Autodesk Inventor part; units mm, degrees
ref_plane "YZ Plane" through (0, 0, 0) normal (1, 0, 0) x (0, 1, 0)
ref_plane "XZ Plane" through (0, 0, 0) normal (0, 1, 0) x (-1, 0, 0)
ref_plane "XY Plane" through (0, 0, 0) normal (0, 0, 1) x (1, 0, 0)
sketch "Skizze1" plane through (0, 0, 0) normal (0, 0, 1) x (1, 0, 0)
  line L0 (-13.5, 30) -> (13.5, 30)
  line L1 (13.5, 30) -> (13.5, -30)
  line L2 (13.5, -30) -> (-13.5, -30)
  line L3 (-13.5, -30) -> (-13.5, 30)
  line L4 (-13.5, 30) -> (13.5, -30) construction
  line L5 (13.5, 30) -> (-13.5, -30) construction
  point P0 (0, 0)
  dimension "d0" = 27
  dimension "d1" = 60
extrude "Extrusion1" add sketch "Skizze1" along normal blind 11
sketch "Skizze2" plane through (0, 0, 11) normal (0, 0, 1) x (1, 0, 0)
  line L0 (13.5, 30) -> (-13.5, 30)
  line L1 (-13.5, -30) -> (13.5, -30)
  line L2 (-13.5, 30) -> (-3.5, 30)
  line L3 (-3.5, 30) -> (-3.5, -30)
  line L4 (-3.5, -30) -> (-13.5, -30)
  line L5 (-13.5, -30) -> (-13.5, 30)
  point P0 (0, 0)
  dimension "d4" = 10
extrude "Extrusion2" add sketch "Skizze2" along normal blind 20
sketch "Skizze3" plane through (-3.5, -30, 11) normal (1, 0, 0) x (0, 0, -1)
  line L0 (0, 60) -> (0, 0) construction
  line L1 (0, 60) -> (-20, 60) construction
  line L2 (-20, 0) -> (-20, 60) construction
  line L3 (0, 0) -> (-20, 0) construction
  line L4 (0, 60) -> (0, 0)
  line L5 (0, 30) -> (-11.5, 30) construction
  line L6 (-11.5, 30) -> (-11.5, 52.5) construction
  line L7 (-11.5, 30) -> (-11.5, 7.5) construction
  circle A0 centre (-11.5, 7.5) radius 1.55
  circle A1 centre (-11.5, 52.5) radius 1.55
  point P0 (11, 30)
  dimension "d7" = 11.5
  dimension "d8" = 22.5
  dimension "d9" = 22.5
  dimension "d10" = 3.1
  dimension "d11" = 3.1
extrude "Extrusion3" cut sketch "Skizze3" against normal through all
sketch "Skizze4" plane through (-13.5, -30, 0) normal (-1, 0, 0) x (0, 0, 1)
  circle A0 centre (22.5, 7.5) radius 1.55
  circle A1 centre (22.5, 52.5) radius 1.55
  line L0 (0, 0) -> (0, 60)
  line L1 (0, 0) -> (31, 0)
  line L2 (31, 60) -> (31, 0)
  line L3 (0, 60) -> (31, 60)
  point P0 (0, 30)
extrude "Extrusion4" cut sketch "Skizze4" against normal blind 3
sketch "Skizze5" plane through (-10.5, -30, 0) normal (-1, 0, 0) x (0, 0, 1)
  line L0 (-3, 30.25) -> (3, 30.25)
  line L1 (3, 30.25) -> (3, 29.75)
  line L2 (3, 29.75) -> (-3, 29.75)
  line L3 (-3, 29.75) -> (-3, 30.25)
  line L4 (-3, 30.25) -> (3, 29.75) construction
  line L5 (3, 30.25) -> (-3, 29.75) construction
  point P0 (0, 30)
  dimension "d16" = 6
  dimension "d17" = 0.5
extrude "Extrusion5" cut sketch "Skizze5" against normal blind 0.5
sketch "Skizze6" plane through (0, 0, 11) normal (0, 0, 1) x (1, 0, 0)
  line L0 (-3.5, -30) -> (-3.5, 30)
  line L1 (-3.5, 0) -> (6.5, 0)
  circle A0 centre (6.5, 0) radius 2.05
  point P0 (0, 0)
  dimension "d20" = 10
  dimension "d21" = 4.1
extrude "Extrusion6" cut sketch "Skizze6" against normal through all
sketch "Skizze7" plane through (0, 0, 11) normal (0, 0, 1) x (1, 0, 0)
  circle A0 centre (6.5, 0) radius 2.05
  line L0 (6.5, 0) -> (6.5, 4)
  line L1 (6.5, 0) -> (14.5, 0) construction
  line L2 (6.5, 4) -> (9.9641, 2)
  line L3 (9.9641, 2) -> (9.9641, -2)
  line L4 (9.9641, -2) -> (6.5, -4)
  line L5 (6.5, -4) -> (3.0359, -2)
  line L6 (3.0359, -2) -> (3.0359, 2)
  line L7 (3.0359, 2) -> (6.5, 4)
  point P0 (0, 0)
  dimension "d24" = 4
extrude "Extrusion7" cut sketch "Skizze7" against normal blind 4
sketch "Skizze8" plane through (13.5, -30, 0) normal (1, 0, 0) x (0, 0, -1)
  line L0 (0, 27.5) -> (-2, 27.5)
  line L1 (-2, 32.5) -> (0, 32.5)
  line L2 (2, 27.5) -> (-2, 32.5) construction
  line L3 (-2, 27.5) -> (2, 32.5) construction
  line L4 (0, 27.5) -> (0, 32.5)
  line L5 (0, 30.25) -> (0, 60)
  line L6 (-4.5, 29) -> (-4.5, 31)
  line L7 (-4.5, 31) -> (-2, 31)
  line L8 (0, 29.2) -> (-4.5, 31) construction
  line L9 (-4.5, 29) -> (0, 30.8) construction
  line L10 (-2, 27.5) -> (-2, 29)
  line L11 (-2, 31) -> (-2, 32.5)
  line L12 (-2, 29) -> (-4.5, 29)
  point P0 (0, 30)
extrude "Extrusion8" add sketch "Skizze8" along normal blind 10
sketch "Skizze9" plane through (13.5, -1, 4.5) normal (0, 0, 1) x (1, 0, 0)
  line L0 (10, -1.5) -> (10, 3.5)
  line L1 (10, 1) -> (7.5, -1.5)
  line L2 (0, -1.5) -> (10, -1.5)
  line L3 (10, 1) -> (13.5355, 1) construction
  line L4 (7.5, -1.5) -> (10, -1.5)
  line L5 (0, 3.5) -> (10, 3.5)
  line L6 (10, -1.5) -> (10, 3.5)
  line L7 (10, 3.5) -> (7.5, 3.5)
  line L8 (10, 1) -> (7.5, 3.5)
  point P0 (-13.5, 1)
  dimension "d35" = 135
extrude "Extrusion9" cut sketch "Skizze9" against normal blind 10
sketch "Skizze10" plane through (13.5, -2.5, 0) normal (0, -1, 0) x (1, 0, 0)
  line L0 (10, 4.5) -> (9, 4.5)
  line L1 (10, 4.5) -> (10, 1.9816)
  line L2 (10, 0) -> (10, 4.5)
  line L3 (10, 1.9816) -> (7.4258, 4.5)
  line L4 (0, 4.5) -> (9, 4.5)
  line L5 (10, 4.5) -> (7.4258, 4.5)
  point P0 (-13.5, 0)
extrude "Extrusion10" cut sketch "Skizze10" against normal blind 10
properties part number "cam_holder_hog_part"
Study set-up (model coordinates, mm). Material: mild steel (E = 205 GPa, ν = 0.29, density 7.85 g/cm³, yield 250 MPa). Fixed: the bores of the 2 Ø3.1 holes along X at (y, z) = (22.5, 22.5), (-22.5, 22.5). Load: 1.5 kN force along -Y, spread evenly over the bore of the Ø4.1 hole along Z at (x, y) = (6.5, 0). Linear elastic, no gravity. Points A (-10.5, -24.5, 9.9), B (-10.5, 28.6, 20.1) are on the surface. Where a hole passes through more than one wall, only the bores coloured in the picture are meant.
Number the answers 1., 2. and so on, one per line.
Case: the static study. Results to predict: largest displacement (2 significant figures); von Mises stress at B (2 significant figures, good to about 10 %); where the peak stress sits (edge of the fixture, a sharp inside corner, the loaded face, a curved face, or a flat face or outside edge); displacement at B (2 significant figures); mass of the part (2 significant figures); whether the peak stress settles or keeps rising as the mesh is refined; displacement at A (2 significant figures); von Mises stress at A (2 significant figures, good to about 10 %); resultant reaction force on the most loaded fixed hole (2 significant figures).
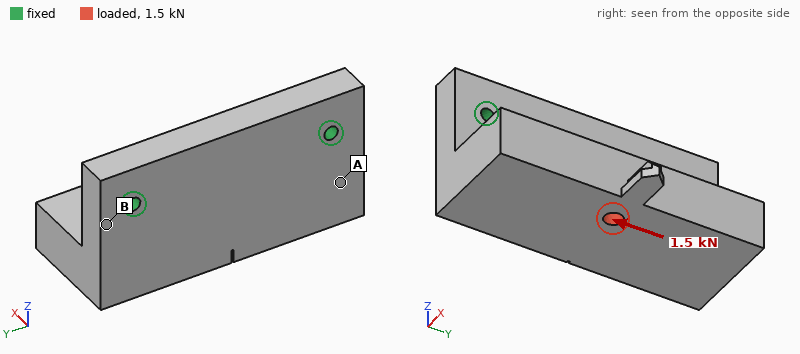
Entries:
1. 5.5 µm
2. 15 MPa
3. edge of the fixture
4. 1.1 µm
5. 190 g
6. keeps rising
7. 2.5 µm
8. 6.9 MPa
9. 1.1 kN
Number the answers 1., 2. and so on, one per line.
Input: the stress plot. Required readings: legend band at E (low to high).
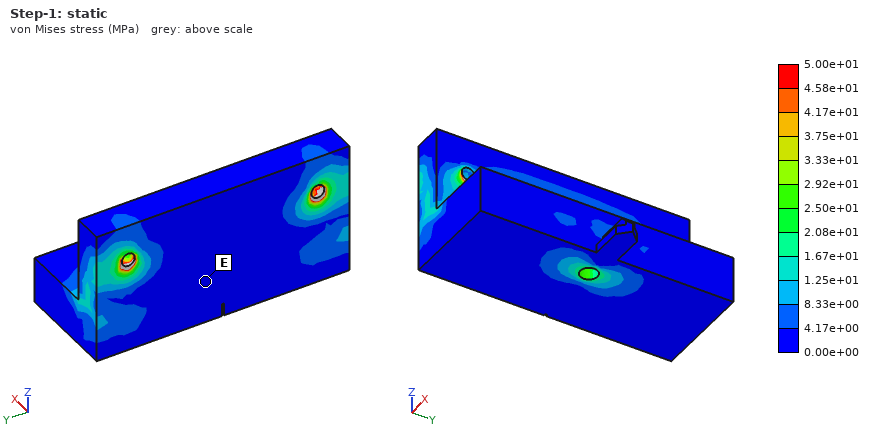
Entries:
1. 0.00e+00 to 4.17e+00 MPa
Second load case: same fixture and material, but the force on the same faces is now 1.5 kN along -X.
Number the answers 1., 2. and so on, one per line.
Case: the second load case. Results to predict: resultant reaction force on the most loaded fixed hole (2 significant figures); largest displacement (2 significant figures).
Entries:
1. 750 N
2. 45 µm
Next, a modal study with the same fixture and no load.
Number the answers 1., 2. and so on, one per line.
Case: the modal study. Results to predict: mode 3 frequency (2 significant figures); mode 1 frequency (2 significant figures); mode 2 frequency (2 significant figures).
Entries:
1. 12 kHz
2. 3500 Hz
3. 7800 Hz
